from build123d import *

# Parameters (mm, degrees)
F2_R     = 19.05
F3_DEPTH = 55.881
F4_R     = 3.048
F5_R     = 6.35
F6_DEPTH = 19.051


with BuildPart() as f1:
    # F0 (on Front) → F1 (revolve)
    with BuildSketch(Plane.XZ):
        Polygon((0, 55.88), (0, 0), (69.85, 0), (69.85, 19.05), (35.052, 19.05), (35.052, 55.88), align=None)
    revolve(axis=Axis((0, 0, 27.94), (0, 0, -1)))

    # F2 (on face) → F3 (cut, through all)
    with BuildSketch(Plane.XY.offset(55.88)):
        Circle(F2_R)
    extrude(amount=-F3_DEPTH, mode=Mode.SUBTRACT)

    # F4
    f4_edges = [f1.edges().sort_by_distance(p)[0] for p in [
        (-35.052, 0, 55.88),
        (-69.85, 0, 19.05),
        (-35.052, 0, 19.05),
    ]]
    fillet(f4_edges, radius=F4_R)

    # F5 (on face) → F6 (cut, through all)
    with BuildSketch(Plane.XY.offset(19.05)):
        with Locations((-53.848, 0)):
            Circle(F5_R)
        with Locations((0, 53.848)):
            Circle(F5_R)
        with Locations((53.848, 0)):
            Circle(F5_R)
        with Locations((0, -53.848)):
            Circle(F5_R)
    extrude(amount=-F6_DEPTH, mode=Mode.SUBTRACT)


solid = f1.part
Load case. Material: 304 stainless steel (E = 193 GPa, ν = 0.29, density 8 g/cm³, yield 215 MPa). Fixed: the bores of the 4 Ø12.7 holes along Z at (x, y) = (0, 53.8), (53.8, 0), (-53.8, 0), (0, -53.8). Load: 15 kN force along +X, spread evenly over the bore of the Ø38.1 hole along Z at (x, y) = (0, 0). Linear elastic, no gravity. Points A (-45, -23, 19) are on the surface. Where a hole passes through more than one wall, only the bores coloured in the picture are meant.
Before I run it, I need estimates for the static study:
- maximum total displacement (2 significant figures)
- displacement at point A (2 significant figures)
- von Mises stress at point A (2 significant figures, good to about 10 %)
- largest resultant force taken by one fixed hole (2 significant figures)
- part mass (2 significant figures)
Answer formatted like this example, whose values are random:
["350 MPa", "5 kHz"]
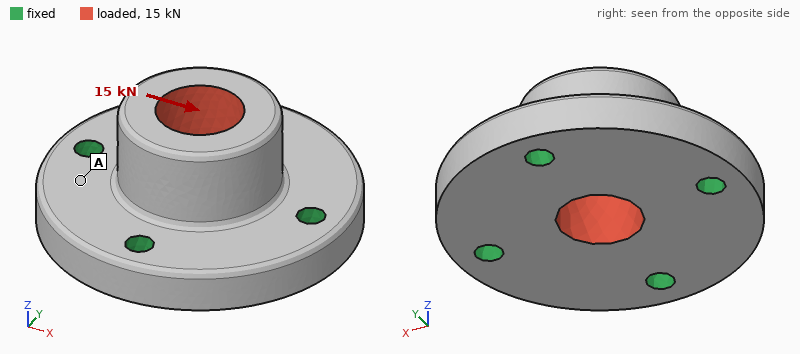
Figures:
["4.8 µm", "0.88 µm", "3.1 MPa", "5.4 kN", "2.9 kg"]
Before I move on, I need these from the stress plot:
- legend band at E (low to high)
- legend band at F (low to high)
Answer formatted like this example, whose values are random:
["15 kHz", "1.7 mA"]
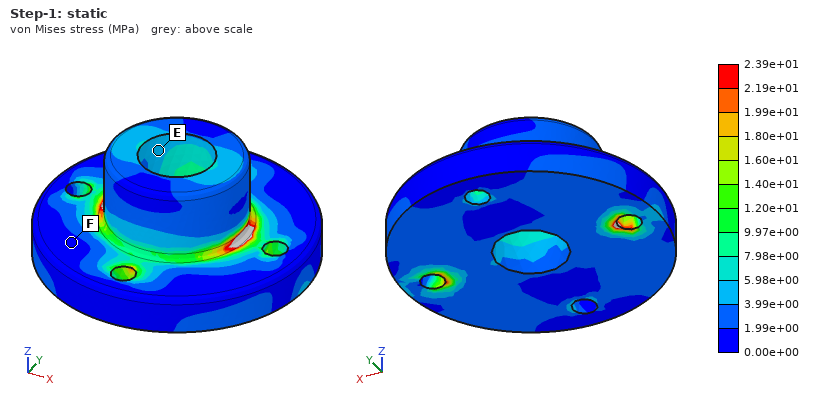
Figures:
["3.99e+00 to 5.98e+00 MPa", "0.00e+00 to 1.99e+00 MPa"]
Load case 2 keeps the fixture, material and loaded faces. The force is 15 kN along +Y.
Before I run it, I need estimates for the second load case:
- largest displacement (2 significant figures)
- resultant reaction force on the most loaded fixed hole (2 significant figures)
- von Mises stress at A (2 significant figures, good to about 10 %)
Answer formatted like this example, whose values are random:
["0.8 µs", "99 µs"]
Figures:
["4.8 µm", "5.4 kN", "2.0 MPa"]
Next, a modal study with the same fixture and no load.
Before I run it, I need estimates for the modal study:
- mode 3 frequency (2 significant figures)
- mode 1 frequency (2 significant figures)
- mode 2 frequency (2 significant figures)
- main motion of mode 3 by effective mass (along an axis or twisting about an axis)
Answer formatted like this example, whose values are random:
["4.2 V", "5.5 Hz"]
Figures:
["9300 Hz", "8600 Hz", "8600 Hz", "along Z"]
